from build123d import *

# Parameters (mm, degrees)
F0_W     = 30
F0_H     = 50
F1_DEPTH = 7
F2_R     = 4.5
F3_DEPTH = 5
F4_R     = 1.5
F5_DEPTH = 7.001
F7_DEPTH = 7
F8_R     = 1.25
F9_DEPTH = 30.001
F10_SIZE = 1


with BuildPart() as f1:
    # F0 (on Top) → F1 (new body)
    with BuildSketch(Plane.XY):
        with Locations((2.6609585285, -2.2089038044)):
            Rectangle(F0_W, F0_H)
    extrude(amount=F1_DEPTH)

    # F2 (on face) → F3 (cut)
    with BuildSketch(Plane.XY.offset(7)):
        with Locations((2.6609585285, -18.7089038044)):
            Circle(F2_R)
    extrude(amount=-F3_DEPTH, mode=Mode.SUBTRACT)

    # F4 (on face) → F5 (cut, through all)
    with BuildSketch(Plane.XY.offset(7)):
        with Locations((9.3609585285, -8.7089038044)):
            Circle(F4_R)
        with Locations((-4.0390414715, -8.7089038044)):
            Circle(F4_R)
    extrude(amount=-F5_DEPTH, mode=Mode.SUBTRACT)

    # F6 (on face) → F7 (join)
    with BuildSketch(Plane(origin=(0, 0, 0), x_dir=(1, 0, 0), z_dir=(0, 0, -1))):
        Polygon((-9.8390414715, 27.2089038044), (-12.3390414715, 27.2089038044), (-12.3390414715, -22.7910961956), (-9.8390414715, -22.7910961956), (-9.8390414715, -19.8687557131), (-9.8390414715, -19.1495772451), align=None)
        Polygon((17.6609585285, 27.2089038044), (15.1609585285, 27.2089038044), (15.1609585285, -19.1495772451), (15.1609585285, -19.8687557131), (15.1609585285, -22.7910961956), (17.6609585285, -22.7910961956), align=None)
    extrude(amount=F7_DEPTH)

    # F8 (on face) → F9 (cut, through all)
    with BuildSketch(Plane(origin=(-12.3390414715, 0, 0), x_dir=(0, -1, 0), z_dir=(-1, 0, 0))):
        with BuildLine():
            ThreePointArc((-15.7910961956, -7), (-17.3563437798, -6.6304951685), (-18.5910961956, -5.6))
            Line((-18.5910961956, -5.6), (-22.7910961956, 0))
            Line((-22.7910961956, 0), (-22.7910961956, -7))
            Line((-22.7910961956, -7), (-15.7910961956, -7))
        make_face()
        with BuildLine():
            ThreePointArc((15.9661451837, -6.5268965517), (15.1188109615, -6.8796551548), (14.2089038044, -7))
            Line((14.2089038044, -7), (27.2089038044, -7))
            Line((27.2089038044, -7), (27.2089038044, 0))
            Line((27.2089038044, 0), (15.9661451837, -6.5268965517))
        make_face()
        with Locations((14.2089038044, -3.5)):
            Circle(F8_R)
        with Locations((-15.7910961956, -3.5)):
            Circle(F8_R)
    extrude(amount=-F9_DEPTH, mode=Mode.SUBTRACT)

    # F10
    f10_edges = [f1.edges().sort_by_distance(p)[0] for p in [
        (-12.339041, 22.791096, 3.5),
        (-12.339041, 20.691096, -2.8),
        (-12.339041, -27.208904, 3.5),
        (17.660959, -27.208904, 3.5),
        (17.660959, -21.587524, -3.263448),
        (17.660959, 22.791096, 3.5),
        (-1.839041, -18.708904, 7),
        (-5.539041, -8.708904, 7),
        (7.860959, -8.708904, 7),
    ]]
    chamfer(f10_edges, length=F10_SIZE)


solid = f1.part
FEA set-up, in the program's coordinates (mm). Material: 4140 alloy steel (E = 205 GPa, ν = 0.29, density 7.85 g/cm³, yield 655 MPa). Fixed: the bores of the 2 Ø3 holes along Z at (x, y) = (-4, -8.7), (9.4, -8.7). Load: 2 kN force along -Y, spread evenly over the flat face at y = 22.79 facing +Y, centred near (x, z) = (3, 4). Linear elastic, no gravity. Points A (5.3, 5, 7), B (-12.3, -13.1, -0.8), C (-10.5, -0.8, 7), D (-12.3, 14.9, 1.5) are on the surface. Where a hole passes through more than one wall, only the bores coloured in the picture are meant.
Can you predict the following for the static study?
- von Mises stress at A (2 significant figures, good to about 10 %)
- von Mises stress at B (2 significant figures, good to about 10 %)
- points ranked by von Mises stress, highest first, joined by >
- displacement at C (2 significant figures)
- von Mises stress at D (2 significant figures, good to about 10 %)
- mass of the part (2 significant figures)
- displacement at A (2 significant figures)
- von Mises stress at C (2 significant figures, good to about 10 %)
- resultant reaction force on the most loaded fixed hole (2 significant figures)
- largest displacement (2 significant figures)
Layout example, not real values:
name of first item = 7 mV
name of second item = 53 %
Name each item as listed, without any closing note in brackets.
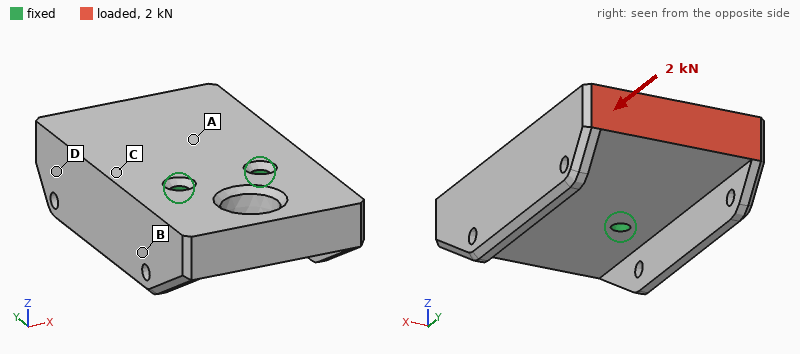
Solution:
von Mises stress at A = 12 MPa
von Mises stress at B = 2.9 MPa
points ranked by von Mises stress, highest first, joined by > = A > C > D > B
displacement at C = 0.74 µm
von Mises stress at D = 5.6 MPa
mass of the part = 89 g
displacement at A = 1.0 µm
von Mises stress at C = 9.0 MPa
resultant reaction force on the most loaded fixed hole = 1.0 kN
largest displacement = 2.5 µm
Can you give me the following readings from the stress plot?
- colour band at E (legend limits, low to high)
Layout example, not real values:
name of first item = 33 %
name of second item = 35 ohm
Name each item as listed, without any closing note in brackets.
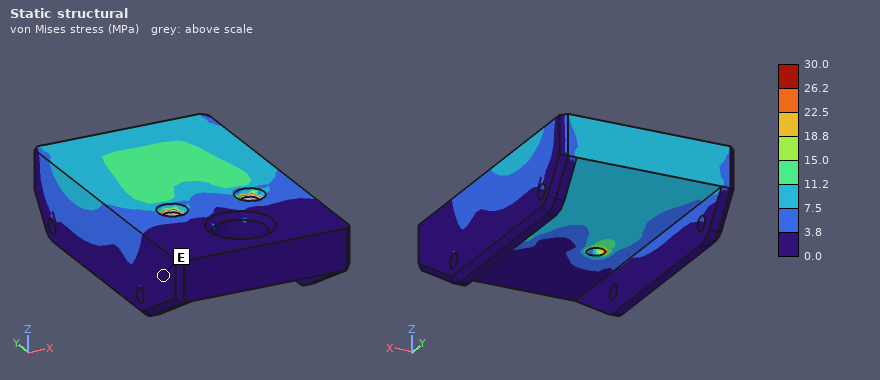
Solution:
colour band at E = 0.0 to 3.8 MPa
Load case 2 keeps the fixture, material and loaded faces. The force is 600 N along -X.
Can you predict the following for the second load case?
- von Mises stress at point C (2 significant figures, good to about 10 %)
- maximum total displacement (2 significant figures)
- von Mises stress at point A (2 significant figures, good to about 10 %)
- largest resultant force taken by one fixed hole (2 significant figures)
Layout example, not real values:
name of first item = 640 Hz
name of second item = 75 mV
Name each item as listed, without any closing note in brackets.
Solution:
von Mises stress at point C = 9.5 MPa
maximum total displacement = 5.2 µm
von Mises stress at point A = 7.6 MPa
largest resultant force taken by one fixed hole = 1.3 kN
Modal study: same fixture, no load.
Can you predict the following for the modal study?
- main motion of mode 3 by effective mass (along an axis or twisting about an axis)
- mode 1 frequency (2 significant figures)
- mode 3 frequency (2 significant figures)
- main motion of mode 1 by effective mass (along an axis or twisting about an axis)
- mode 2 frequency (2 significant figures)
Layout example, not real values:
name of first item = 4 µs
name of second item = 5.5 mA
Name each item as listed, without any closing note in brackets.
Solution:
main motion of mode 3 by effective mass = along X
mode 1 frequency = 5500 Hz
mode 3 frequency = 12 kHz
main motion of mode 1 by effective mass = along Z
mode 2 frequency = 11 kHz
